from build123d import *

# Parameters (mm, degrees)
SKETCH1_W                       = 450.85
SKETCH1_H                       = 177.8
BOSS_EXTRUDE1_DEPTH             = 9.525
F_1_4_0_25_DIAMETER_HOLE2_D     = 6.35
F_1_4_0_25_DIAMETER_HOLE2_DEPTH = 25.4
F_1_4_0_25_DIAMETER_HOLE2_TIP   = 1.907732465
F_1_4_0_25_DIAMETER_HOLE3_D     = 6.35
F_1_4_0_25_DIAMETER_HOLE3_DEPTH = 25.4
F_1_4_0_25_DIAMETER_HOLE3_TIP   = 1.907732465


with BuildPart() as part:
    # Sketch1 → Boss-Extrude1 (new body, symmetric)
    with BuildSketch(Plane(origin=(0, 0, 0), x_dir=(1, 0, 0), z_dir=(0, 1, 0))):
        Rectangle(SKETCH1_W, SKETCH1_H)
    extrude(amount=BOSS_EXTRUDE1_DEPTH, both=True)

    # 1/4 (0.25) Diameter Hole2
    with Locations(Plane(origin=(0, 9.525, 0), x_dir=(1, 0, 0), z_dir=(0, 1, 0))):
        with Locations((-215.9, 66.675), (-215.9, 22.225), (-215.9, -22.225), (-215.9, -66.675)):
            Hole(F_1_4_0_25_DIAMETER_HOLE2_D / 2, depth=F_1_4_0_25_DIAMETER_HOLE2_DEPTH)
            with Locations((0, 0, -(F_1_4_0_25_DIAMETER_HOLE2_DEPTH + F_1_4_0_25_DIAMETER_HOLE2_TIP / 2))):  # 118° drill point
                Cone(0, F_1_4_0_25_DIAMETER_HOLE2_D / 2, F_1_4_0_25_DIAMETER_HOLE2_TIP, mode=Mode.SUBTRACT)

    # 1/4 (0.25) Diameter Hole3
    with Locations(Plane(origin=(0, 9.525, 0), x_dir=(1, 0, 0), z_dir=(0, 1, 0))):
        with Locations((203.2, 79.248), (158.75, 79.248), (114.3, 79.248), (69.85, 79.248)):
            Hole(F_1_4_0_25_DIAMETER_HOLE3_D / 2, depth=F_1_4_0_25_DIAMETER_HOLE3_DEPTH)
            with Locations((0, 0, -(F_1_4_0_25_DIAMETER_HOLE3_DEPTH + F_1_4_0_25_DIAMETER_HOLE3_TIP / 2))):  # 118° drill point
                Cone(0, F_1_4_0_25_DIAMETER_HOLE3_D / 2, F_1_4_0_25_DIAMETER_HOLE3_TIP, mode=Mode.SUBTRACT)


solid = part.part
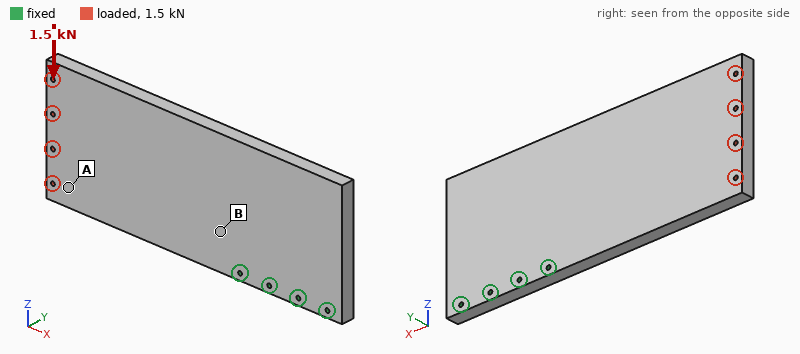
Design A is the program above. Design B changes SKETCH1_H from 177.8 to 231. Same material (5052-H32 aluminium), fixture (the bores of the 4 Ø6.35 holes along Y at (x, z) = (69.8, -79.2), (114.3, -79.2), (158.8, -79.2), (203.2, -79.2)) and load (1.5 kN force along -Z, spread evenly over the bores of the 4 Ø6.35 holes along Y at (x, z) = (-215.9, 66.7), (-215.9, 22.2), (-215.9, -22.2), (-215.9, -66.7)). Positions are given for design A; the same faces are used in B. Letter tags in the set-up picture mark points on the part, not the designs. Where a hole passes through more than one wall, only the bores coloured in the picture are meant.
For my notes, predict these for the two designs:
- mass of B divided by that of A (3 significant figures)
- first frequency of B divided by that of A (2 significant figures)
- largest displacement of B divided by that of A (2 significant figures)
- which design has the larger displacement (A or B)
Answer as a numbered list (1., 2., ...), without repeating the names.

1. 1.30
2. 0.99
3. 0.71
4. A
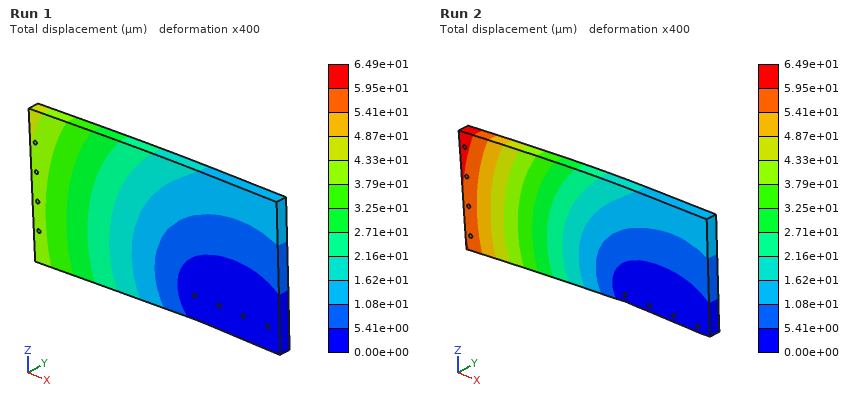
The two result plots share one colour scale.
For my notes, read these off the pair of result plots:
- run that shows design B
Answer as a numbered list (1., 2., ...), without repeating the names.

1. Run 1
